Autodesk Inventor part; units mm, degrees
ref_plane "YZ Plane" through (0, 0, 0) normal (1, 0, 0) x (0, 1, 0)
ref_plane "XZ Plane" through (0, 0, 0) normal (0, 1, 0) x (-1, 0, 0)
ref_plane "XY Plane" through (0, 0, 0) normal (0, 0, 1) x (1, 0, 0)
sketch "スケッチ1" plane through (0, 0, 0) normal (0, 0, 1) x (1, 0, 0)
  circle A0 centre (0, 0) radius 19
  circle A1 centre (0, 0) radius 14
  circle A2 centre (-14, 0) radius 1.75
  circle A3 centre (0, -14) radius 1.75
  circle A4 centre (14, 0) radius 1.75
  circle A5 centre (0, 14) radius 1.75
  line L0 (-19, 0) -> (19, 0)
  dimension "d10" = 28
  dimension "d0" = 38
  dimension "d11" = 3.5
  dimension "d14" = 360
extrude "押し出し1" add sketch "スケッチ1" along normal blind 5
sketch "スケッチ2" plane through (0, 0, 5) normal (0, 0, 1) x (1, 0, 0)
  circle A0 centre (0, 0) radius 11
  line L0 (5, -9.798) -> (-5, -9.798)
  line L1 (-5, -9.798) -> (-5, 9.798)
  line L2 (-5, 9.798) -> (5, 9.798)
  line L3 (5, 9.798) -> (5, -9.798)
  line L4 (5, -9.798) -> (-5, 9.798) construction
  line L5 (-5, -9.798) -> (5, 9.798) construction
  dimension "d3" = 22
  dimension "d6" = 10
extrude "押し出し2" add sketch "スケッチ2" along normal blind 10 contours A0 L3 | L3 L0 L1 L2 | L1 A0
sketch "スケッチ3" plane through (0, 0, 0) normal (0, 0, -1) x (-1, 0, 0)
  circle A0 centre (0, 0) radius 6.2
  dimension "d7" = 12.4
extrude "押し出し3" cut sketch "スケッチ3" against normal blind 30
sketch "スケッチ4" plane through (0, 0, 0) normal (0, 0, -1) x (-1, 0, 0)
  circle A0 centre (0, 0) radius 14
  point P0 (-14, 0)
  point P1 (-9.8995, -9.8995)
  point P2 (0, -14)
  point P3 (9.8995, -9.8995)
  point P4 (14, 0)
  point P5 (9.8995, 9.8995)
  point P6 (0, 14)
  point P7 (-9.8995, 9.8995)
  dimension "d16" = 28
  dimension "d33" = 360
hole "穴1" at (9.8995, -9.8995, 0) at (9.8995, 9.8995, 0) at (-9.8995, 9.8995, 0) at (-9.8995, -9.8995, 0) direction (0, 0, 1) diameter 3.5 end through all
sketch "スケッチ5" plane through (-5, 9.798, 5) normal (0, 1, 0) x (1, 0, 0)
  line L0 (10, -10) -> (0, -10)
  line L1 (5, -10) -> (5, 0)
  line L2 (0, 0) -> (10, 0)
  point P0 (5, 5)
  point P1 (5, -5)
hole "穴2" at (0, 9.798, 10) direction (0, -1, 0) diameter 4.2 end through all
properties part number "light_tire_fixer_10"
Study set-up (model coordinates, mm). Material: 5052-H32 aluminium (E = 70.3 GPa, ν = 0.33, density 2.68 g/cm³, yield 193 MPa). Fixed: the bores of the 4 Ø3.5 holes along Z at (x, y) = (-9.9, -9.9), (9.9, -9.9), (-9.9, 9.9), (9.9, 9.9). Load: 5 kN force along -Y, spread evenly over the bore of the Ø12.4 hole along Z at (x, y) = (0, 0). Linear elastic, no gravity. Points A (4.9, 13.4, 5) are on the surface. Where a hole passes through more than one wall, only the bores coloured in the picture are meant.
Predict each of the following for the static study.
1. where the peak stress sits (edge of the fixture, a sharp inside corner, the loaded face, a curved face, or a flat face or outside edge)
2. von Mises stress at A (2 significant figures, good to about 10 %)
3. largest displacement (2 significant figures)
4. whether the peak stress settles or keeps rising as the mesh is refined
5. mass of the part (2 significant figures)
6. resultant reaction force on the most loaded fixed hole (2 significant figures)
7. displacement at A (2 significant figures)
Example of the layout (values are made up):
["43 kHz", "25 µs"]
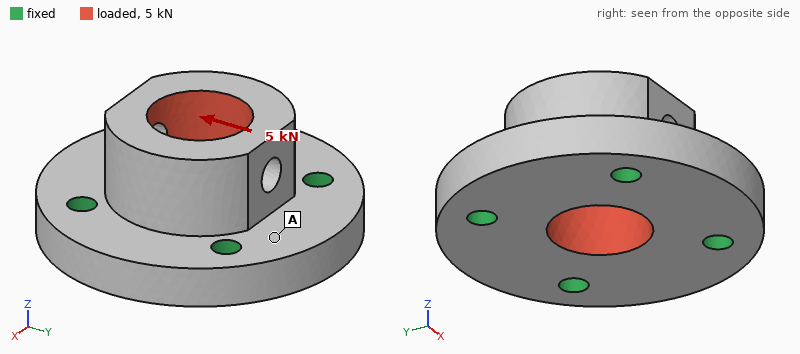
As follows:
["a sharp inside corner", "13 MPa", "13 µm", "keeps rising", "19 g", "1.4 kN", "2.8 µm"]
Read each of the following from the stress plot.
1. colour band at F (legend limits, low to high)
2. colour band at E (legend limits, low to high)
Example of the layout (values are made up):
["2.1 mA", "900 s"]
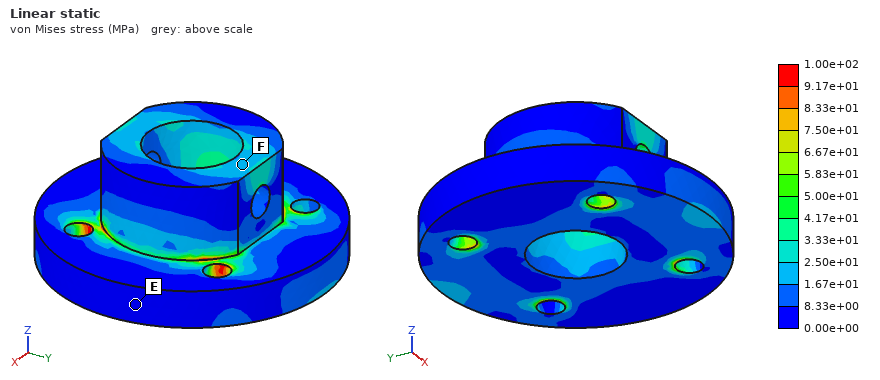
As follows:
["1.67e+01 to 2.50e+01 MPa", "0.00e+00 to 8.33e+00 MPa"]
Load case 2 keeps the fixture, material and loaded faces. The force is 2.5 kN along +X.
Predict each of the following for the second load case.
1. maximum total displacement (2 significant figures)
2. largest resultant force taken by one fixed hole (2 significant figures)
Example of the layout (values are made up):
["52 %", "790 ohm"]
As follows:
["7.4 µm", "700 N"]
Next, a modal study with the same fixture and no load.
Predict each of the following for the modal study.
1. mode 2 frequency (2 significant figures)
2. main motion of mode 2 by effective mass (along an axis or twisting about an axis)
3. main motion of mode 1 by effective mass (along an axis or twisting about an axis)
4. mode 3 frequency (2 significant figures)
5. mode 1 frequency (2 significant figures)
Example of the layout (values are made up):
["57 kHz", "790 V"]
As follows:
["36 kHz", "along Y", "along X", "38 kHz", "33 kHz"]
